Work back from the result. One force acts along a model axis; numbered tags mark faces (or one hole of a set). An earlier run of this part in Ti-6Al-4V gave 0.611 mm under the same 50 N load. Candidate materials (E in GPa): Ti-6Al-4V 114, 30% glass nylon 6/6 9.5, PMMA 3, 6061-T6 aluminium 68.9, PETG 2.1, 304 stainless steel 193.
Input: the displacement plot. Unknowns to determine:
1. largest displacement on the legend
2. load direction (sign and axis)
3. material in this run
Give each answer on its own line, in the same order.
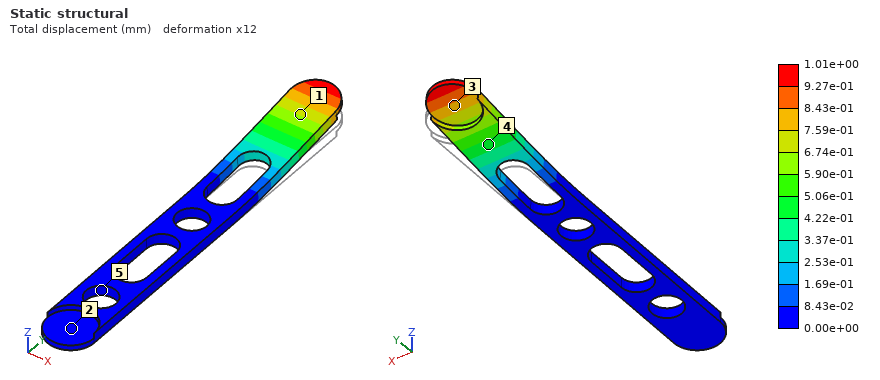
1.01e+00 mm
+Z
6061-T6 aluminium
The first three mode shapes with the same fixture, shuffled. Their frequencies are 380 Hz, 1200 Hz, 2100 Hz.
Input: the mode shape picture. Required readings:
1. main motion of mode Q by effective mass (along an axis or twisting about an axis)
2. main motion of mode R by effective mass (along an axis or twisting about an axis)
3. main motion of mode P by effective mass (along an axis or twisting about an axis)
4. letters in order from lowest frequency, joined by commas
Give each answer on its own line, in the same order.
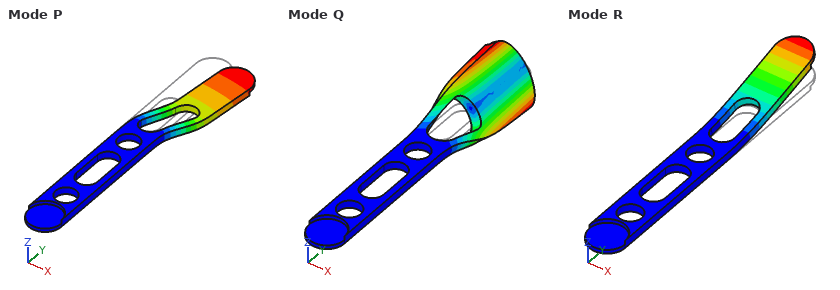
twisting about Y
along Z
along X
R, P, Q
